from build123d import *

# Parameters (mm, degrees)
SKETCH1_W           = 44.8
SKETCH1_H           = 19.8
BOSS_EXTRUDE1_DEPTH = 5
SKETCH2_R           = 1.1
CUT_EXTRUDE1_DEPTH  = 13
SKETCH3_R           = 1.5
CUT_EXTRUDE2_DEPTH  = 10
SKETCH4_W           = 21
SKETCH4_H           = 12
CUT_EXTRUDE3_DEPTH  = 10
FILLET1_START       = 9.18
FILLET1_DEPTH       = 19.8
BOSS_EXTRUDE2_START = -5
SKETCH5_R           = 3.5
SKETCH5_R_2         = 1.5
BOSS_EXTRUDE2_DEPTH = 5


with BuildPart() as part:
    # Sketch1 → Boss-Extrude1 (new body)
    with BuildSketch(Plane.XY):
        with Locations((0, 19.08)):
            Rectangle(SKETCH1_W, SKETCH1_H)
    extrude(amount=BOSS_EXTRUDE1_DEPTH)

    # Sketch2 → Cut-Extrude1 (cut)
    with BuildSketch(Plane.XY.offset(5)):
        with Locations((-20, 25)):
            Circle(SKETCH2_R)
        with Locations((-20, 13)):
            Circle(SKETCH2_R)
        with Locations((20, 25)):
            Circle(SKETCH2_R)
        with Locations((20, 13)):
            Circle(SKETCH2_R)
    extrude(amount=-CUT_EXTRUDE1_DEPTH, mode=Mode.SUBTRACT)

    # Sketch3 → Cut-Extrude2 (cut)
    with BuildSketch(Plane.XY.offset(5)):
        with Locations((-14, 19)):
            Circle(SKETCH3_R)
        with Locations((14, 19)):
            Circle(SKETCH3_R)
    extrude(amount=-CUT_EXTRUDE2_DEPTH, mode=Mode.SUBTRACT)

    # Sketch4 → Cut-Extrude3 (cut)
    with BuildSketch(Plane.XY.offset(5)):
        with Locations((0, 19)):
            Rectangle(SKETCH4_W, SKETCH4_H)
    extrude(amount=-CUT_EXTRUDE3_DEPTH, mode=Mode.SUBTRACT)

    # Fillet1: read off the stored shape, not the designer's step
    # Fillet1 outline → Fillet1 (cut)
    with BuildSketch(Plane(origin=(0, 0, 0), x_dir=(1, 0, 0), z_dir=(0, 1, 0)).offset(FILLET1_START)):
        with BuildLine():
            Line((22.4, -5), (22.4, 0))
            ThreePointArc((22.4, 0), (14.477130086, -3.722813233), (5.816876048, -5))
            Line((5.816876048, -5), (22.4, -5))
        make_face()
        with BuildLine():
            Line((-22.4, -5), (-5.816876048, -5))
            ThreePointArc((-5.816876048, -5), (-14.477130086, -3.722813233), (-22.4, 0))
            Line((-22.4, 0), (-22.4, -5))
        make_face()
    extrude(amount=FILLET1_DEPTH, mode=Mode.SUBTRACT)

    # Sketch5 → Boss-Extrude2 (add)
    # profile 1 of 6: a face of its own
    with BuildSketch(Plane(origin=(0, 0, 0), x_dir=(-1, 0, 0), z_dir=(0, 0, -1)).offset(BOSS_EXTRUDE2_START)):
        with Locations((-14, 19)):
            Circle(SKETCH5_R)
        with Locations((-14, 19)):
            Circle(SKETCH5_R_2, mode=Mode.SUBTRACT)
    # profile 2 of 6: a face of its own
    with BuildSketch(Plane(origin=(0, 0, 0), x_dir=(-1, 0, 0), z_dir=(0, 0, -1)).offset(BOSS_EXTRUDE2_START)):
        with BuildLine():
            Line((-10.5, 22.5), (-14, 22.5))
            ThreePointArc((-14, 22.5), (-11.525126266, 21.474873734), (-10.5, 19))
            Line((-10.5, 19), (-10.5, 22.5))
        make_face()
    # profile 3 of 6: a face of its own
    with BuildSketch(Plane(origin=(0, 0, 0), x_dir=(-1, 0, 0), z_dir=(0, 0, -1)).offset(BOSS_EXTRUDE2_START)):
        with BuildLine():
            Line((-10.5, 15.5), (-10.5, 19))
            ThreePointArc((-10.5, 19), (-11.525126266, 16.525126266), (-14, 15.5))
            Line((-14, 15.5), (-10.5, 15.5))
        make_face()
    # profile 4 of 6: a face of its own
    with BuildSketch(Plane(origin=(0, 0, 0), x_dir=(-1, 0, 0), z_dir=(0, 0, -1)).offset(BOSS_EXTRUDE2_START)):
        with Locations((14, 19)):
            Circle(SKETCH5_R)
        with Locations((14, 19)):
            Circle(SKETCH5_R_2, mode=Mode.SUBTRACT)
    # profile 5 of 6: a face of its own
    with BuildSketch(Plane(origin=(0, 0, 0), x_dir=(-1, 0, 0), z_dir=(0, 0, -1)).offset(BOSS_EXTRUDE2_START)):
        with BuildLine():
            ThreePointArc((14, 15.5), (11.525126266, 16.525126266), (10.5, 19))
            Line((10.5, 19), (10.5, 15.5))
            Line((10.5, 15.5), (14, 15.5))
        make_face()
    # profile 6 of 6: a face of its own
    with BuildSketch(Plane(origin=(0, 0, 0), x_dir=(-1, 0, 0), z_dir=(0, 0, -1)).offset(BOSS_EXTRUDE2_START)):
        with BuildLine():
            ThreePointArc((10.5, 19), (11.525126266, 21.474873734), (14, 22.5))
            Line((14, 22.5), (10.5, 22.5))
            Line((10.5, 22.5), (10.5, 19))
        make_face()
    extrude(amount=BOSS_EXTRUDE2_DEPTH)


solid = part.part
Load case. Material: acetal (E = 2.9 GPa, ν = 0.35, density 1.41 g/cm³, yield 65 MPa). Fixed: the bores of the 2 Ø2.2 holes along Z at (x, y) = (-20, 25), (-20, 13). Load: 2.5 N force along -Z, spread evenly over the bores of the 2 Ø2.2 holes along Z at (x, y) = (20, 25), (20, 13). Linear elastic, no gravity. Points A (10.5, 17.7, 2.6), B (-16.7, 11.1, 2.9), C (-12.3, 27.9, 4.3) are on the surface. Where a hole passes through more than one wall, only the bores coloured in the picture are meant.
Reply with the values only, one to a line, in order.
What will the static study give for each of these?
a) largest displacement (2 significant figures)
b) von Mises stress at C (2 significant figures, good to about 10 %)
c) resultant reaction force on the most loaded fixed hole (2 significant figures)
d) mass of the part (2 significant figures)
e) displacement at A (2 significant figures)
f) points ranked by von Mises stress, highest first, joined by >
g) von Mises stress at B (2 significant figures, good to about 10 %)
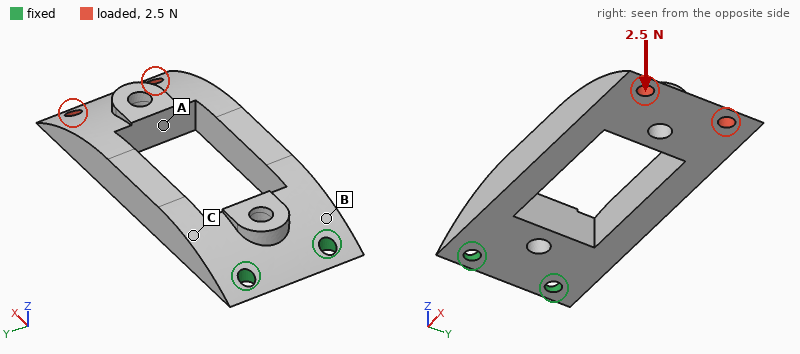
0.56 mm
2.4 MPa
1.3 N
3.0 g
0.36 mm
B > C > A
3.7 MPa
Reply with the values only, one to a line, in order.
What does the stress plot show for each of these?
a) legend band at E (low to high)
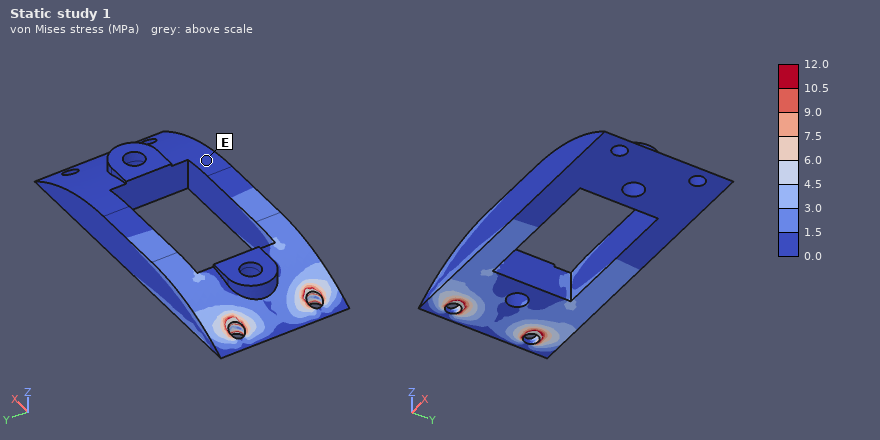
0.0 to 1.5 MPa
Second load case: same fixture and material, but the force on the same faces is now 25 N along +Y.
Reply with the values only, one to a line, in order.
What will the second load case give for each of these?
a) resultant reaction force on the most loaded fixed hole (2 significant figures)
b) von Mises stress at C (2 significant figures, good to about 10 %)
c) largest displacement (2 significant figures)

75 N
6.8 MPa
0.51 mm
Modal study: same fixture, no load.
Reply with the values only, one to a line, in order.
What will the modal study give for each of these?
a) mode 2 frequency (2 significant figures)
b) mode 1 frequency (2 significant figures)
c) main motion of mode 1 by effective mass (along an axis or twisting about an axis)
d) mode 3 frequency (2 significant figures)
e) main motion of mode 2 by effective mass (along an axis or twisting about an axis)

1100 Hz
370 Hz
along Z
1500 Hz
along Y
